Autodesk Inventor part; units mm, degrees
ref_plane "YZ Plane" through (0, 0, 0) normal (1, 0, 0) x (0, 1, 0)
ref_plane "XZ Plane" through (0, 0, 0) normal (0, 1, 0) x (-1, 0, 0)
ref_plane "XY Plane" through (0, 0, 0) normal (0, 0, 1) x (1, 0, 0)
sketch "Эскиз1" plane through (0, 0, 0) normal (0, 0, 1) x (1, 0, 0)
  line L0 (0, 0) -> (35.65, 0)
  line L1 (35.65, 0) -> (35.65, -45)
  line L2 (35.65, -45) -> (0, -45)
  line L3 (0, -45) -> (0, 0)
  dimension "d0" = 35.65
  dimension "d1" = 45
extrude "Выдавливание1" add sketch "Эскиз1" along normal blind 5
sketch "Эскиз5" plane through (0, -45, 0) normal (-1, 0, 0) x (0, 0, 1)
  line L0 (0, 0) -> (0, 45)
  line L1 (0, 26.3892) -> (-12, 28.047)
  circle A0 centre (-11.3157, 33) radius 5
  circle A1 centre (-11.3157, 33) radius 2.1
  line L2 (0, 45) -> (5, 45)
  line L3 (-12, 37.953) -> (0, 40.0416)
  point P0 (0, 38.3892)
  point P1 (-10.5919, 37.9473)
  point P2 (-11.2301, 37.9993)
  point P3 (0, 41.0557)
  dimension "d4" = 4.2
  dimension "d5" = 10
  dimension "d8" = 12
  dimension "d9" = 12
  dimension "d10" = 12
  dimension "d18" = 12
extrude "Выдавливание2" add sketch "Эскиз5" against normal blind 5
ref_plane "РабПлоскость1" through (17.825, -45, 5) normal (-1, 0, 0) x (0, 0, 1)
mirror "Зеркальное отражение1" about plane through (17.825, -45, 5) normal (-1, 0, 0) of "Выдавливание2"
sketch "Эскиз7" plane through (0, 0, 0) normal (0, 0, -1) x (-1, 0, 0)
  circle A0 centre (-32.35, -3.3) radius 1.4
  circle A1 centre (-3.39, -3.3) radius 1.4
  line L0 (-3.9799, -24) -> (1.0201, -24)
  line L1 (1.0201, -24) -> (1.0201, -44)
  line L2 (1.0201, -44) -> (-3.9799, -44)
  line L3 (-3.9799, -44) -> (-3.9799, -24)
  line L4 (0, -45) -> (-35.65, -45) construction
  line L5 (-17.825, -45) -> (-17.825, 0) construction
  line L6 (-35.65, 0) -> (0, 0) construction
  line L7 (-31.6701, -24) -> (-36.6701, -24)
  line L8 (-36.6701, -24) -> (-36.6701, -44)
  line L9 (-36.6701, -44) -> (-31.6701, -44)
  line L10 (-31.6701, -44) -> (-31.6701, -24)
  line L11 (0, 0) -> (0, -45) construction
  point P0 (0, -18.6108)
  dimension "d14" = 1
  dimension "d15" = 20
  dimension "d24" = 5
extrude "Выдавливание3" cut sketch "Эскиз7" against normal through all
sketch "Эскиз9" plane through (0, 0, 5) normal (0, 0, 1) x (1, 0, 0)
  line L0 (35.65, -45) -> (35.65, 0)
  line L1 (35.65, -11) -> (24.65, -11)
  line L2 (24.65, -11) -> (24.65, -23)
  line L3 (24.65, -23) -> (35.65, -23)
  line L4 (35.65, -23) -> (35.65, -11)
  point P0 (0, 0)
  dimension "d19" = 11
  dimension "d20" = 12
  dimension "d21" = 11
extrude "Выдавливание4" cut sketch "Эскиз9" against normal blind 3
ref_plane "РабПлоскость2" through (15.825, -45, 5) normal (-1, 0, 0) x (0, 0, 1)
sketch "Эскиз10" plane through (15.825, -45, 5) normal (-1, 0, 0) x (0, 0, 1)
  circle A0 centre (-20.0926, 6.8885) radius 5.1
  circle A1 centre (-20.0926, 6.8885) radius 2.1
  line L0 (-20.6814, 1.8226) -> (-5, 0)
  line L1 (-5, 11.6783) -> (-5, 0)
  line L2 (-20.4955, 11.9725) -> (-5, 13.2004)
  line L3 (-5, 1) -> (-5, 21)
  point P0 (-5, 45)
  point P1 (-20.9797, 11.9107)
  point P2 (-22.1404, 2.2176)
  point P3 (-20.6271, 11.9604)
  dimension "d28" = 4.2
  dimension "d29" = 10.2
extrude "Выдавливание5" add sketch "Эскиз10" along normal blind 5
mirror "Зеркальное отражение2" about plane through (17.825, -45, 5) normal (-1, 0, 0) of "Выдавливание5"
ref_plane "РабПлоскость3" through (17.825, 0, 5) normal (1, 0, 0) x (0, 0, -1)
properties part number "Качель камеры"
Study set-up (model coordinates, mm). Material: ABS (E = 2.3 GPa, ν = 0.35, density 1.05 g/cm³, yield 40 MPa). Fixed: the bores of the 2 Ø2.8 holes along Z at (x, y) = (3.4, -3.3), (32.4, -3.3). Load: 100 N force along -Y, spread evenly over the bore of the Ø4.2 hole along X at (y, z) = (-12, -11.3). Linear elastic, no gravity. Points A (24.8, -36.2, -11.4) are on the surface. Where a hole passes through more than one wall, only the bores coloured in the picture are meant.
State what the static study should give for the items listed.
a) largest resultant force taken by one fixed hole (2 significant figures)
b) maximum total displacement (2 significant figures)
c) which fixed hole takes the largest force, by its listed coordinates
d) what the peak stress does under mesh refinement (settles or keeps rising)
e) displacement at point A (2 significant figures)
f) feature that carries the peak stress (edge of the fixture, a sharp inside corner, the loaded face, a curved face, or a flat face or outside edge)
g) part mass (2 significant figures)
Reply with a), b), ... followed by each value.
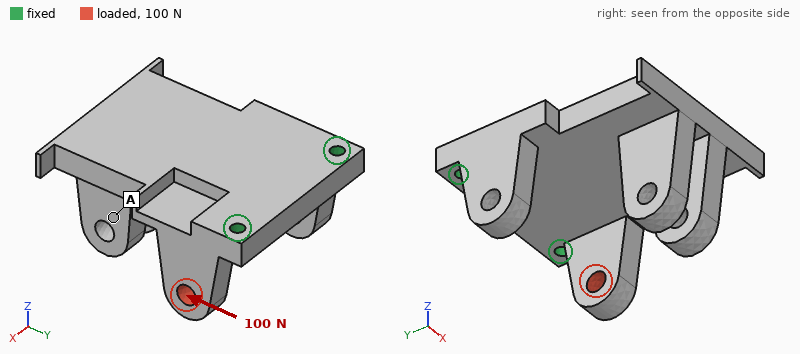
a) 100 N
b) 0.65 mm
c) (32.4, -3.3)
d) keeps rising
e) 0.48 mm
f) edge of the fixture
g) 11 g
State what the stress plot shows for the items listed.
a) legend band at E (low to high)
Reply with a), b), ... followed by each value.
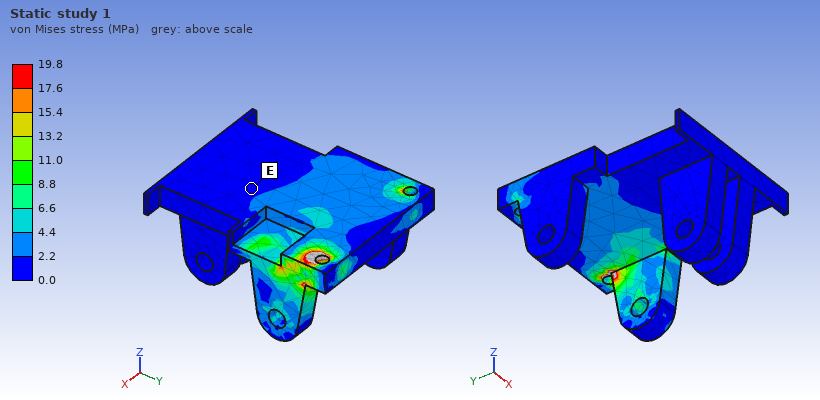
a) 0.0 to 2.2 MPa
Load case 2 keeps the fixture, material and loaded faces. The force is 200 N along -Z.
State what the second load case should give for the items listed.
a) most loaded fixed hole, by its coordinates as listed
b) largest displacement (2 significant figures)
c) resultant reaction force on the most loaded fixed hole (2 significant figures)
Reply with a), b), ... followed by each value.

a) (32.4, -3.3)
b) 0.64 mm
c) 200 N
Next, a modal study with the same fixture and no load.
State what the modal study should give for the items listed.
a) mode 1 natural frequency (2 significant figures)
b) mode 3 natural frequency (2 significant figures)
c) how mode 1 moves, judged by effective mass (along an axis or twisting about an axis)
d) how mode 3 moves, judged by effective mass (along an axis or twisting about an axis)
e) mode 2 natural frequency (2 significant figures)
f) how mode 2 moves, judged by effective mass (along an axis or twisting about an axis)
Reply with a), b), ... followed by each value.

a) 470 Hz
b) 2000 Hz
c) along Z
d) along Z
e) 1200 Hz
f) along X
